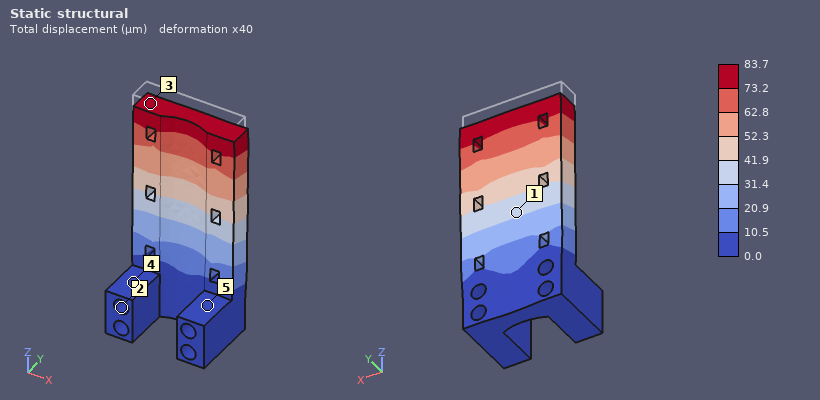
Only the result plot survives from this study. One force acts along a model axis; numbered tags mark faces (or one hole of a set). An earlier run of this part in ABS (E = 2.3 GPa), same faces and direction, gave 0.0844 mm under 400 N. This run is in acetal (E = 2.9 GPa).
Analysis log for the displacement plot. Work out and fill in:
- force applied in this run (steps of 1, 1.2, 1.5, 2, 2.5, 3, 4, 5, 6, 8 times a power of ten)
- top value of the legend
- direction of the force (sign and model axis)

500 N
83.7 µm
-Z
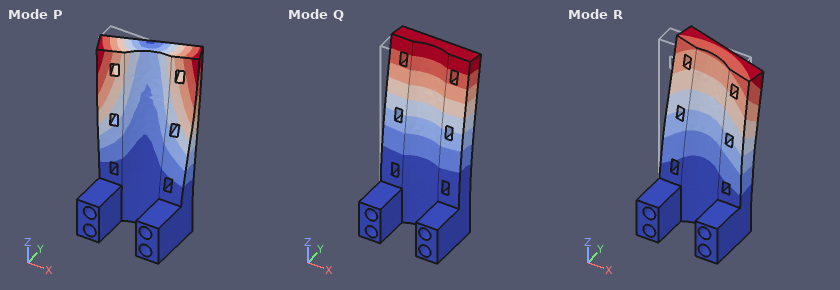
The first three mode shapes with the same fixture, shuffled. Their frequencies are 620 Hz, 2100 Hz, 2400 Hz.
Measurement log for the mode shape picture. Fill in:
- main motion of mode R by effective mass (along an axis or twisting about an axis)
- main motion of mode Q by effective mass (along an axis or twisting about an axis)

along X
along Y
